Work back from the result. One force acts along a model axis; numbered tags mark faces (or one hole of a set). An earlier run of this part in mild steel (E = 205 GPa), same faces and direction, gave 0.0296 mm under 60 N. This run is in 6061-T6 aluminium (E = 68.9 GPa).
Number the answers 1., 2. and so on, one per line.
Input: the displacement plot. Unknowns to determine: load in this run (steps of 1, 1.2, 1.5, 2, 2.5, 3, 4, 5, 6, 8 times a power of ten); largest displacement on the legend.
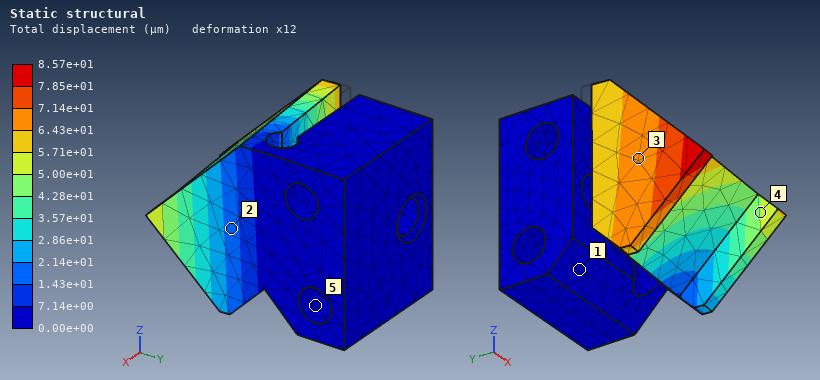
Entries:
1. 60 N
2. 8.57e+01 µm
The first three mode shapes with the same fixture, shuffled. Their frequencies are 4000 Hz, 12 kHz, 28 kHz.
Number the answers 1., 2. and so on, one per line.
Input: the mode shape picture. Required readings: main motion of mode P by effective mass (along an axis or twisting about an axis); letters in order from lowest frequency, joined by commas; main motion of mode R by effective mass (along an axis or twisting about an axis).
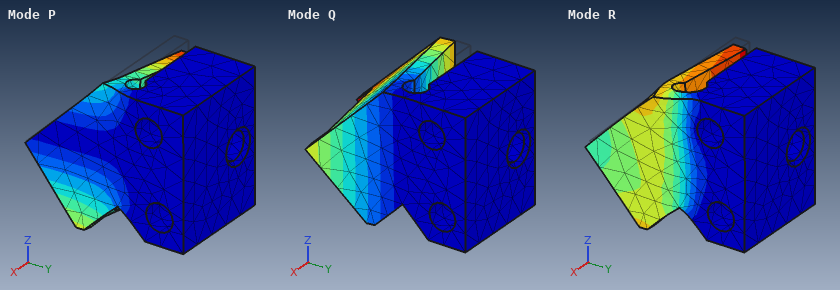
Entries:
1. along Z
2. Q, P, R
3. along X
